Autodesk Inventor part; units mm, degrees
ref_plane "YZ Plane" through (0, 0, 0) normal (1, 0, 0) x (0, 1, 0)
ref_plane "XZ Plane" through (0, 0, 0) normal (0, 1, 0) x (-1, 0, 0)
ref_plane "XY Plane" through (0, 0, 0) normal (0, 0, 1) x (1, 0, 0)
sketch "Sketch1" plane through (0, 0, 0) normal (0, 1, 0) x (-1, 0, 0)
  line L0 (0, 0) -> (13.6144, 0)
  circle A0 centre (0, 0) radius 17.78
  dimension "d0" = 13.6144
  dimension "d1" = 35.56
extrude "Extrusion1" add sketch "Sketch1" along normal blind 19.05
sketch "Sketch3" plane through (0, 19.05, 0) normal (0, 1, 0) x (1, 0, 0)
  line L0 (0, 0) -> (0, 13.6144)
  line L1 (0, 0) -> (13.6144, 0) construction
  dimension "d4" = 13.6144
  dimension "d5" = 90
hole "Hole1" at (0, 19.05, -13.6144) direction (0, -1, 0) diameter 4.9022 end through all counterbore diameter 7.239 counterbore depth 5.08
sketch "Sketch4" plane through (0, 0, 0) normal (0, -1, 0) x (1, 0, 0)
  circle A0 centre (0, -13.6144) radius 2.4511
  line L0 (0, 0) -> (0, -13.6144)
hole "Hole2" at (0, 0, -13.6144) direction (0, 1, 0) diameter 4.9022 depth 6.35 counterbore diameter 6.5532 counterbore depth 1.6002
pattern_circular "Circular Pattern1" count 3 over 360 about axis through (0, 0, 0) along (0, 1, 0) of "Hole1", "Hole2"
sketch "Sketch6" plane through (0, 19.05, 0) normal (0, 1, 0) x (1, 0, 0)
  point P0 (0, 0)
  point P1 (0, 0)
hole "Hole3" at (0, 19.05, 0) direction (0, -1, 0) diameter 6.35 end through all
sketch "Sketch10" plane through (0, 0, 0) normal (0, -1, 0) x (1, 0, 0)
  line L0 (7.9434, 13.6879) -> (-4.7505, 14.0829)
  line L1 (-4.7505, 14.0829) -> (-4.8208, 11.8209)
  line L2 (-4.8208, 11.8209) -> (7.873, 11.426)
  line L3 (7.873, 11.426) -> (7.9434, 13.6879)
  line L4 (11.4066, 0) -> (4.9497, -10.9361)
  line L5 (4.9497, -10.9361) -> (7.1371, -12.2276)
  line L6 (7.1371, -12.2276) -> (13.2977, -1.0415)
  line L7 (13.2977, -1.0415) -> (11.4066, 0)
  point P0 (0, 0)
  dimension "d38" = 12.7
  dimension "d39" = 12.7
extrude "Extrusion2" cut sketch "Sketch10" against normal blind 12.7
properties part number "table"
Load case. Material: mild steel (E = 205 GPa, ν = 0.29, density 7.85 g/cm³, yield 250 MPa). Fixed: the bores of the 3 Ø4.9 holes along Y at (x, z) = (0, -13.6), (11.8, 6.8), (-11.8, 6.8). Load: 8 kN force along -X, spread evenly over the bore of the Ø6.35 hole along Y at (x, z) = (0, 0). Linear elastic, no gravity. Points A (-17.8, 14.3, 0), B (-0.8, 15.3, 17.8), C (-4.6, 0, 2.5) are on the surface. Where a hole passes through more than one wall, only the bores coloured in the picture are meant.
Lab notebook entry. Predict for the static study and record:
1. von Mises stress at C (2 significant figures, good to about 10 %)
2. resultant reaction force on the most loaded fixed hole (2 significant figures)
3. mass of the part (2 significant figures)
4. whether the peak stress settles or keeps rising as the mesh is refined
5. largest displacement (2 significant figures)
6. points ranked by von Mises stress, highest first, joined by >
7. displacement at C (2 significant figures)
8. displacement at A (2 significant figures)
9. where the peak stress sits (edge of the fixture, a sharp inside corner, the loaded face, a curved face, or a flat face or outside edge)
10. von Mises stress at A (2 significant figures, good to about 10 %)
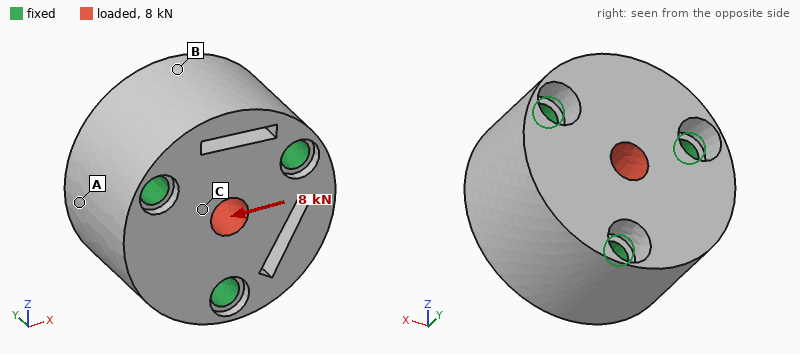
20 MPa
2.9 kN
130 g
keeps rising
1.6 µm
C > A > B
0.77 µm
0.78 µm
edge of the fixture
9.3 MPa
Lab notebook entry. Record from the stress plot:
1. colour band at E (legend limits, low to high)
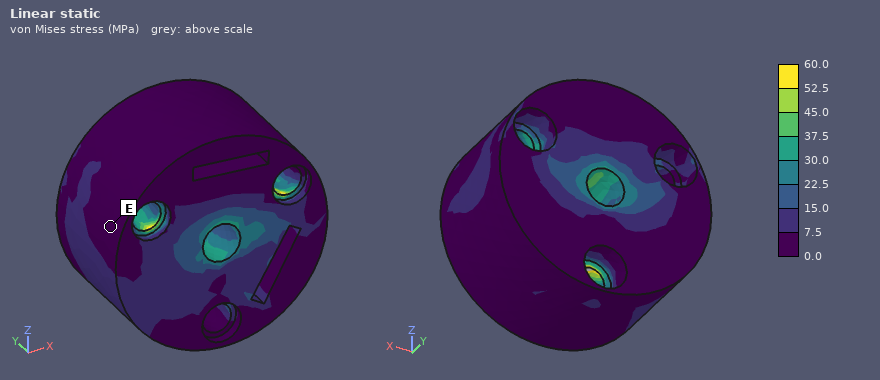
0.0 to 7.5 MPa
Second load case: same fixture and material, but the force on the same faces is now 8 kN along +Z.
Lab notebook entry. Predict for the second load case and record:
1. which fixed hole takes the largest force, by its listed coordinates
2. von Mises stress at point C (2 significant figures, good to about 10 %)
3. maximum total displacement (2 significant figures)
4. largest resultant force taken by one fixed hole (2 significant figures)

(0, -13.6)
13 MPa
1.8 µm
3.1 kN
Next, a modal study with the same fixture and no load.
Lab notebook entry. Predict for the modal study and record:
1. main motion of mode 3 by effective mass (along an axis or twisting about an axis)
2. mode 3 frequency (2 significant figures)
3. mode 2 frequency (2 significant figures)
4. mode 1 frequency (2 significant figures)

along Y
46 kHz
39 kHz
39 kHz
